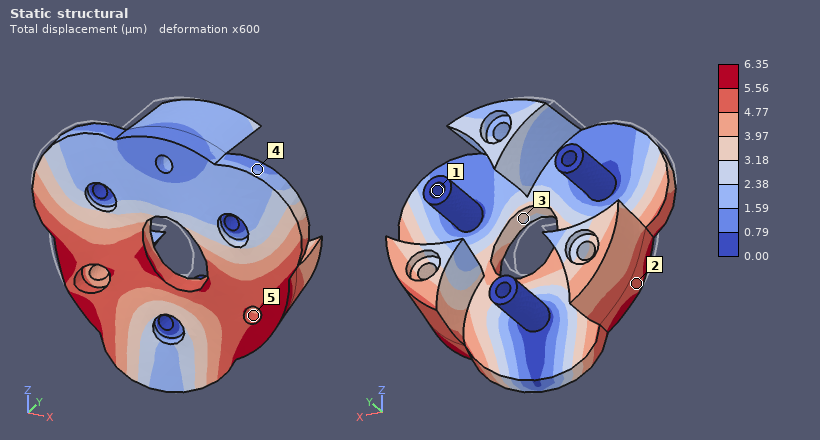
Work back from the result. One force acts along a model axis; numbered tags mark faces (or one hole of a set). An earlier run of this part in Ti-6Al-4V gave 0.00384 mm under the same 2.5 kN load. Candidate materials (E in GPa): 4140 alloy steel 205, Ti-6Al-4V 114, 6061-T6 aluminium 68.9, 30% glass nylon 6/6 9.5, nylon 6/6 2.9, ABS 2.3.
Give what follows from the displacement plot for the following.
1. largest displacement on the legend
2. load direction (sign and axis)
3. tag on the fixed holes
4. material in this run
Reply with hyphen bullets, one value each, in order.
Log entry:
- 6.35 µm
- +X
- 1
- 6061-T6 aluminium
